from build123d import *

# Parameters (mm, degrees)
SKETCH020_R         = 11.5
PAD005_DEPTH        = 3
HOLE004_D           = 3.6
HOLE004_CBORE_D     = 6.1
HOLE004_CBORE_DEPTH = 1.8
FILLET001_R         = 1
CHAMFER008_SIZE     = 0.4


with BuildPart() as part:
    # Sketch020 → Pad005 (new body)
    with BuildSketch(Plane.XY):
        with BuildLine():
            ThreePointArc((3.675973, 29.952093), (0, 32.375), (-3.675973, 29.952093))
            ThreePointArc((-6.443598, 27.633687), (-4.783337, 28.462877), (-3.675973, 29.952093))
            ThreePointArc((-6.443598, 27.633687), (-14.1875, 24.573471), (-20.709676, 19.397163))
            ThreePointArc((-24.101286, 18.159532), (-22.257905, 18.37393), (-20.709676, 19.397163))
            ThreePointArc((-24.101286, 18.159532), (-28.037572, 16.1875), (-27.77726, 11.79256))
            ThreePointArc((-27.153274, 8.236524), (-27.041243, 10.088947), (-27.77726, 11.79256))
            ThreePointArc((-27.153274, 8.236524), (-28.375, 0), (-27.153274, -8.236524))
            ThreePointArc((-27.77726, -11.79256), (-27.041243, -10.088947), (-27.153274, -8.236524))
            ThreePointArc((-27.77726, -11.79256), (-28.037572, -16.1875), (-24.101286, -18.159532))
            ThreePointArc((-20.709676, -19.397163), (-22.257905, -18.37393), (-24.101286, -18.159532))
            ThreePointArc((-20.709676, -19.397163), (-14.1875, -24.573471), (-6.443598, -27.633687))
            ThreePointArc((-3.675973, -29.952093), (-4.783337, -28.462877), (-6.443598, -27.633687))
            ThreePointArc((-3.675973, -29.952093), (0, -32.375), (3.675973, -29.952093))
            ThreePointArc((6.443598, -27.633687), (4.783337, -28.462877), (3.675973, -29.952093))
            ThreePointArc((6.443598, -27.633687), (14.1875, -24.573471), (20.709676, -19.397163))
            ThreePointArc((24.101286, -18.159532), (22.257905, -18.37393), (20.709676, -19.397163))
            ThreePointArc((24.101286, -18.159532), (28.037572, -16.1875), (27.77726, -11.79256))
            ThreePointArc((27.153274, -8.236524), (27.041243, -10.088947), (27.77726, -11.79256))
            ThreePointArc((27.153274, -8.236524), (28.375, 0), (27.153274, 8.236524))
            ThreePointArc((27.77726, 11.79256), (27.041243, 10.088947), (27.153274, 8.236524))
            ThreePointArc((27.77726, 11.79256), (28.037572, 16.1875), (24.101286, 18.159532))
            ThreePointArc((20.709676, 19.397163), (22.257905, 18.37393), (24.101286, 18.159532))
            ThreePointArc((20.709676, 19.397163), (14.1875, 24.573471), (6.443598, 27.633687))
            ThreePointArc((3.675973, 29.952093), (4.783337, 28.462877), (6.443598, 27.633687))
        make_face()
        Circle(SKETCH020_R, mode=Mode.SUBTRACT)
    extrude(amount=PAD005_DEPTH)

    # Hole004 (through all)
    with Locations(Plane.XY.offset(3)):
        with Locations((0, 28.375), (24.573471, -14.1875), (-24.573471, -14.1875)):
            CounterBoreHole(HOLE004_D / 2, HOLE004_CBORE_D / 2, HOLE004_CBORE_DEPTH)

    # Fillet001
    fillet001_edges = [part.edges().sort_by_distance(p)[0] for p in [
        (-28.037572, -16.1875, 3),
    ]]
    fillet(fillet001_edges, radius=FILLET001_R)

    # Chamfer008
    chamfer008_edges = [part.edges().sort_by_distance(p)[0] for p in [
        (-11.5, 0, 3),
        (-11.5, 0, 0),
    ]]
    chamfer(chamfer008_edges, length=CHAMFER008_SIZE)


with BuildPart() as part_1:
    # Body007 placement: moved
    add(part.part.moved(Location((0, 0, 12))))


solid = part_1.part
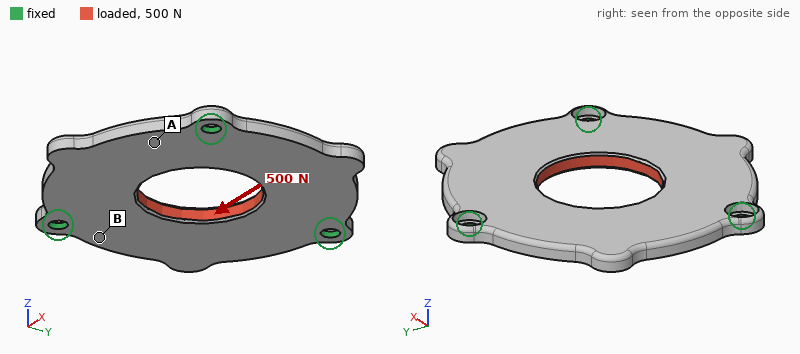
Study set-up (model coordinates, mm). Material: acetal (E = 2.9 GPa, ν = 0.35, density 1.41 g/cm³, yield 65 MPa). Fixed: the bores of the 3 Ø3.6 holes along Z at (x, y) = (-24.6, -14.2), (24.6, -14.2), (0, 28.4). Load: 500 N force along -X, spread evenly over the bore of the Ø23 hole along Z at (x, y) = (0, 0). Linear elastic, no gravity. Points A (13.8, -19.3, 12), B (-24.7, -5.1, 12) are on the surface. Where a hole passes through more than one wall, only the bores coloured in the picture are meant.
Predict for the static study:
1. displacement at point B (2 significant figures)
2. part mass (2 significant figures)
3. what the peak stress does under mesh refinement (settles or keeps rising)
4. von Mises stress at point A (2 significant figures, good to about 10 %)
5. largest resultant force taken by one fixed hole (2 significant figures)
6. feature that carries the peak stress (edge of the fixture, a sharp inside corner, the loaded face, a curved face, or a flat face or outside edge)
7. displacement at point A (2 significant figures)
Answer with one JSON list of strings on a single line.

["0.040 mm", "9.3 g", "keeps rising", "4.5 MPa", "170 N", "edge of the fixture", "0.044 mm"]
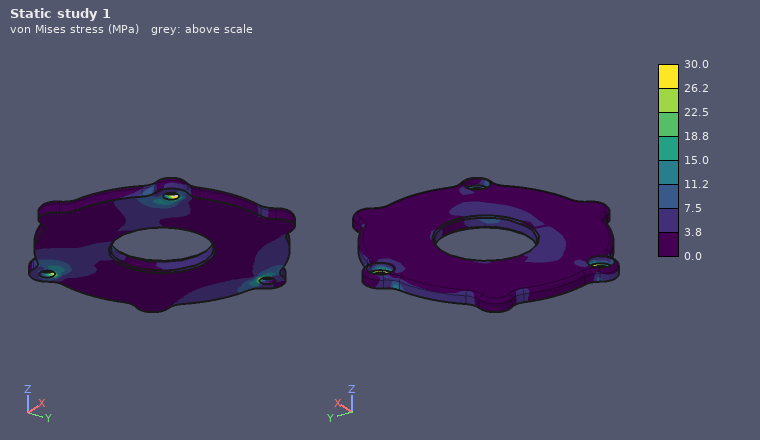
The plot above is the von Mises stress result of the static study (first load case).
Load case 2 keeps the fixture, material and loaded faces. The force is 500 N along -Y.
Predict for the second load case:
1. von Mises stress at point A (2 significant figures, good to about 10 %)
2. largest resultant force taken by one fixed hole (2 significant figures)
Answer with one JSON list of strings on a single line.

["3.3 MPa", "170 N"]
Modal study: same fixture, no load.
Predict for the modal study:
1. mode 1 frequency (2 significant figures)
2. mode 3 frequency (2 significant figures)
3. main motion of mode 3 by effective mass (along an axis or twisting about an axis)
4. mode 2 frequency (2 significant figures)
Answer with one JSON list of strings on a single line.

["1100 Hz", "1300 Hz", "along Z", "1100 Hz"]
